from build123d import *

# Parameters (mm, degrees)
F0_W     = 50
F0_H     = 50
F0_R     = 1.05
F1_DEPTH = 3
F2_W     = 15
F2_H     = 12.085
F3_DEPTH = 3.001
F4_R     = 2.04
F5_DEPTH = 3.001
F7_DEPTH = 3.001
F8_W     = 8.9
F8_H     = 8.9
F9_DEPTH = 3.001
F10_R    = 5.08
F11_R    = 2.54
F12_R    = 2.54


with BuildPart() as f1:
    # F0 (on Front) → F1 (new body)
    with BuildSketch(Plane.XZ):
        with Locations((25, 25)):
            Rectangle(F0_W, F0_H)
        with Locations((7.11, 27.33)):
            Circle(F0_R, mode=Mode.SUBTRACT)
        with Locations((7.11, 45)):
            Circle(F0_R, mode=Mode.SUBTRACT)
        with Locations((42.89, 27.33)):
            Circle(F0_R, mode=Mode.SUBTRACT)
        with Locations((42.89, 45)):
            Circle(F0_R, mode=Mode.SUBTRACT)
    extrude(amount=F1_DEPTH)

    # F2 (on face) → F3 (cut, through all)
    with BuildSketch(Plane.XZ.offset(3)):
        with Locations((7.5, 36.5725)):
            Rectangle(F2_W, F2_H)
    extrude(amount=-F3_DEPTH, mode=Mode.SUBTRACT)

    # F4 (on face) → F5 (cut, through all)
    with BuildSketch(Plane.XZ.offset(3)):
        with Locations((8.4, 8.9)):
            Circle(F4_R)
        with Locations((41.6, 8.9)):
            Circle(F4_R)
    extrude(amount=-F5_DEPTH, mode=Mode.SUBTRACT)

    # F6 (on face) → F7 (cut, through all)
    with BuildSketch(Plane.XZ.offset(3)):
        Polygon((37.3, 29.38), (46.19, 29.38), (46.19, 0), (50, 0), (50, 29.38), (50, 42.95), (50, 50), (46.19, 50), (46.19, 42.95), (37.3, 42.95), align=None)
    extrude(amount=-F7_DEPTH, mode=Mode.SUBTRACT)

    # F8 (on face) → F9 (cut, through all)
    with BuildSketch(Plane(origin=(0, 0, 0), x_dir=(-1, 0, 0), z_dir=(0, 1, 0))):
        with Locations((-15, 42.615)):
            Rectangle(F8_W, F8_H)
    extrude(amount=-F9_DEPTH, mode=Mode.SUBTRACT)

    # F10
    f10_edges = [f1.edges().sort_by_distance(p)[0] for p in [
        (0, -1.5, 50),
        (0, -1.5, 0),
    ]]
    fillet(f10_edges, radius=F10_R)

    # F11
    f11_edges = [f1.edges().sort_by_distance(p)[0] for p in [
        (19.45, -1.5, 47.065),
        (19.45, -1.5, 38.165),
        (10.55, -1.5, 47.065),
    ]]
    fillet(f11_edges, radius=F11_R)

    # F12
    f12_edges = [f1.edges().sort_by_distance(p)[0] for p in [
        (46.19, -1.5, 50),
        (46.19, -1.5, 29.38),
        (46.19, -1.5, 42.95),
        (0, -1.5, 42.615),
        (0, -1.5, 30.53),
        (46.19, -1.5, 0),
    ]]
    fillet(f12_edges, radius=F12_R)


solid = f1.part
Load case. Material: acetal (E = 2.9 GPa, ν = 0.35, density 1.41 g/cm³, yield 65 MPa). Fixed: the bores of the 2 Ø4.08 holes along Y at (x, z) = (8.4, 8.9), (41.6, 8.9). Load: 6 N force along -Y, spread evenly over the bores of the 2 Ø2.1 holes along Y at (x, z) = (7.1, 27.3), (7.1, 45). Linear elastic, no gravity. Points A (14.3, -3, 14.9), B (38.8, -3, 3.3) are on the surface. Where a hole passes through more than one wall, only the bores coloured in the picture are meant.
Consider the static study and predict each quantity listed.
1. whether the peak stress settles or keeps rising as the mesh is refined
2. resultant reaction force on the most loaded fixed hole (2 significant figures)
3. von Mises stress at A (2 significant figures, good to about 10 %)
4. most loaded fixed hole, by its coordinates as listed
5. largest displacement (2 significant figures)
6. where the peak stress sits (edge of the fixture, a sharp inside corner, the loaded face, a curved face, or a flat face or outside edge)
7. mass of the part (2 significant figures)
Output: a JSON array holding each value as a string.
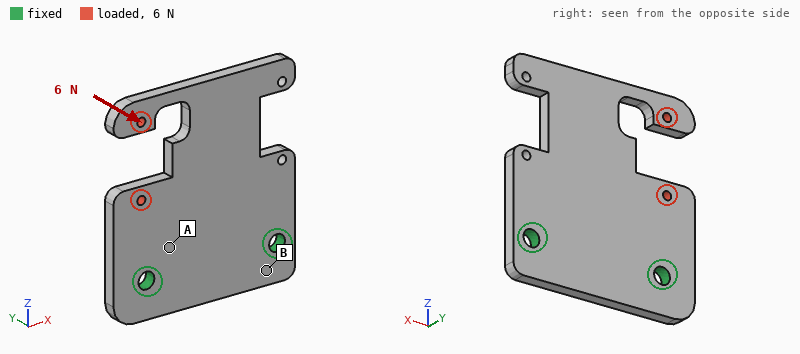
["keeps rising", "6.4 N", "2.2 MPa", "(8.4, 8.9)", "0.80 mm", "edge of the fixture", "8.0 g"]
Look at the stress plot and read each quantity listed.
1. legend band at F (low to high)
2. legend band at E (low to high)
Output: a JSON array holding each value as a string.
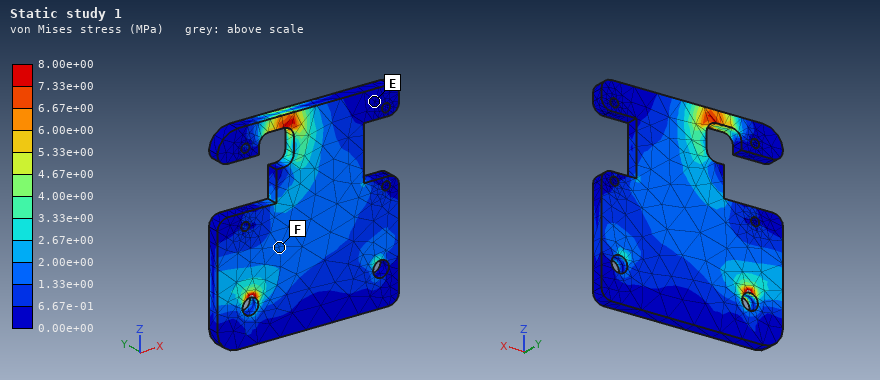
["1.33e+00 to 2.00e+00 MPa", "0.00e+00 to 6.67e-01 MPa"]
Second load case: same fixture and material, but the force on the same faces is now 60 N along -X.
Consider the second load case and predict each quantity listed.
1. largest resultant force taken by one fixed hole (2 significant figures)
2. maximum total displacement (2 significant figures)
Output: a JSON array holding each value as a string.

["57 N", "0.77 mm"]
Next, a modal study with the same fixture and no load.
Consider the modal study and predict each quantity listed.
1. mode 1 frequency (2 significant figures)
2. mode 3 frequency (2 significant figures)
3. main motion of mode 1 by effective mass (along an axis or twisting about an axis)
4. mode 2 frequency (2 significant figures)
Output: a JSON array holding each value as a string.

["420 Hz", "1200 Hz", "along Y", "760 Hz"]
